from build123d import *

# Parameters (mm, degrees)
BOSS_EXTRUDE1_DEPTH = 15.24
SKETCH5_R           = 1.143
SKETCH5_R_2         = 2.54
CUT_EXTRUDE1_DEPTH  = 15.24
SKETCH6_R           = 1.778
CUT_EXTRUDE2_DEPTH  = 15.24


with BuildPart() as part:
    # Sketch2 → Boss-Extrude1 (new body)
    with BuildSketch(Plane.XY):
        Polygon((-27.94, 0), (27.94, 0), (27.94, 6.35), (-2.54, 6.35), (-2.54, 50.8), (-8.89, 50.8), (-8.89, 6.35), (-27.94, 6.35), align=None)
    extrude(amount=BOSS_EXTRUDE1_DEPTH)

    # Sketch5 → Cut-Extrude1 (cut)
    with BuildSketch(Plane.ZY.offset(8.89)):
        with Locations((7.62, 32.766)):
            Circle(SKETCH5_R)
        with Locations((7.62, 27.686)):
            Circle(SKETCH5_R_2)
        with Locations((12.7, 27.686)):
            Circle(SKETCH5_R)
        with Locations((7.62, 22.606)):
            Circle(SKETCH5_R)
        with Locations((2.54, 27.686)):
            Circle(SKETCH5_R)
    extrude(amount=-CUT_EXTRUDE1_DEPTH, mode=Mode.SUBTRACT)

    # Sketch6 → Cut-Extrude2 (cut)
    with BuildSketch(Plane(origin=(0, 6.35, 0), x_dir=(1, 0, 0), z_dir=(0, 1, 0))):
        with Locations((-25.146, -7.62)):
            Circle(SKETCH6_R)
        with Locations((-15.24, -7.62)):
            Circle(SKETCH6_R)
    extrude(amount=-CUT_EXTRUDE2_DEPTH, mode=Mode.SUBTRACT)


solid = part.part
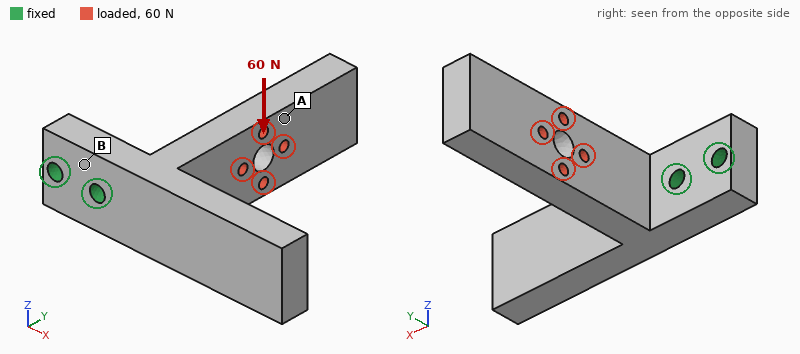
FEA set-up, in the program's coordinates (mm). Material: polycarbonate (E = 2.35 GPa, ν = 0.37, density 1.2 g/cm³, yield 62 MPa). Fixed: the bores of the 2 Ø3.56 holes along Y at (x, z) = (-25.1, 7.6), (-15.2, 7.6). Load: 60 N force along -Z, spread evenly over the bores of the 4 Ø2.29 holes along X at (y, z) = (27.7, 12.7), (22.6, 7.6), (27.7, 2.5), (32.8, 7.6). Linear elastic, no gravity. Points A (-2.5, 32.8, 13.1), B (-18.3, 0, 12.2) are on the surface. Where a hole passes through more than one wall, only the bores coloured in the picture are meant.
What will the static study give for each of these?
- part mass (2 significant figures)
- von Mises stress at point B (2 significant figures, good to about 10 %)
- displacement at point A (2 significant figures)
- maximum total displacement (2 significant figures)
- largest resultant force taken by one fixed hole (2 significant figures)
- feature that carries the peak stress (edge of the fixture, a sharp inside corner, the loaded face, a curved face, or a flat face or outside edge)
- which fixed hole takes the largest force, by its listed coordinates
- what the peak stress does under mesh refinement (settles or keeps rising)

11 g
4.7 MPa
0.48 mm
0.76 mm
93 N
edge of the fixture
(-15.2, 7.6)
keeps rising
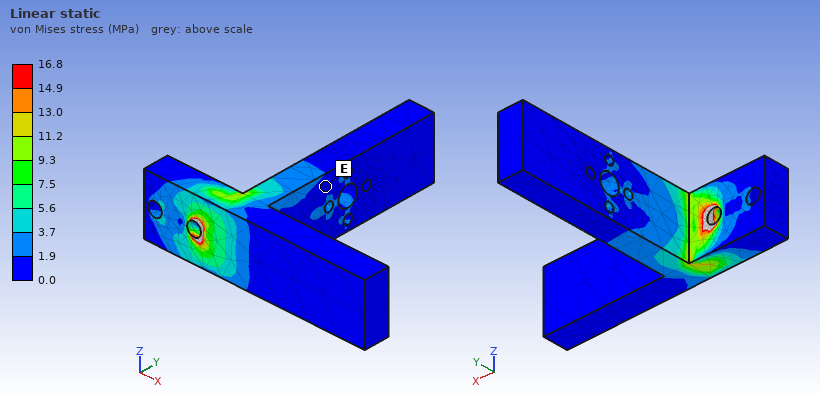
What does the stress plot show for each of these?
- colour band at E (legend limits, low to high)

0.0 to 1.9 MPa
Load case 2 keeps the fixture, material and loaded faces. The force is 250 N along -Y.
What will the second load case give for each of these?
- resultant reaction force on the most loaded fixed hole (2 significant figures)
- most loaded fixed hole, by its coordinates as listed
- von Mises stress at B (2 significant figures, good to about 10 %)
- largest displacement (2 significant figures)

300 N
(-15.2, 7.6)
5.4 MPa
0.79 mm
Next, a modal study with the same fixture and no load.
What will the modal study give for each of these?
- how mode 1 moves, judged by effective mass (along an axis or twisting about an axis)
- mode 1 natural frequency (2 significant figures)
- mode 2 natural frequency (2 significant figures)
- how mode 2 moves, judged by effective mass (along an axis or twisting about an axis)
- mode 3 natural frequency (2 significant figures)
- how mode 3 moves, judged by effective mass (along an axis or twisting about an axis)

along X
460 Hz
740 Hz
along Z
990 Hz
along Y
